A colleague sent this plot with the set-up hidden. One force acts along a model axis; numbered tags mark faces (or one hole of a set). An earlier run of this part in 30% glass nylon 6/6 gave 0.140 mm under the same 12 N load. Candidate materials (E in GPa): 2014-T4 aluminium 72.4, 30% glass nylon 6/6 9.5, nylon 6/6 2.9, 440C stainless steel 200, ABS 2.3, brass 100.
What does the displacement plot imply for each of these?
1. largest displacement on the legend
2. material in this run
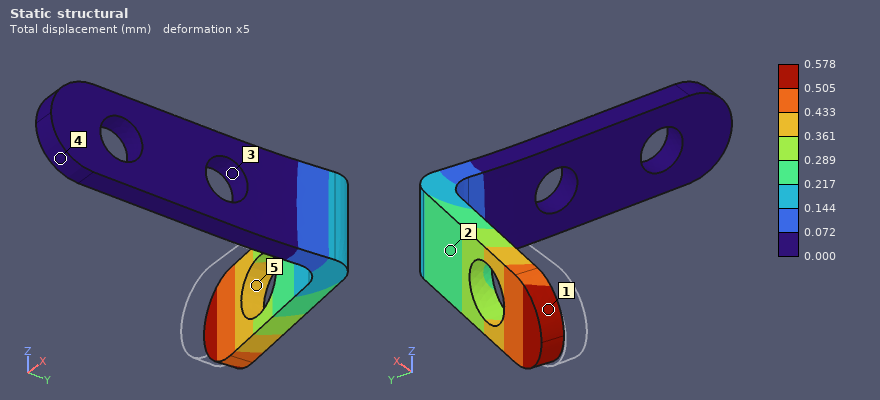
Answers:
0.578 mm
ABS
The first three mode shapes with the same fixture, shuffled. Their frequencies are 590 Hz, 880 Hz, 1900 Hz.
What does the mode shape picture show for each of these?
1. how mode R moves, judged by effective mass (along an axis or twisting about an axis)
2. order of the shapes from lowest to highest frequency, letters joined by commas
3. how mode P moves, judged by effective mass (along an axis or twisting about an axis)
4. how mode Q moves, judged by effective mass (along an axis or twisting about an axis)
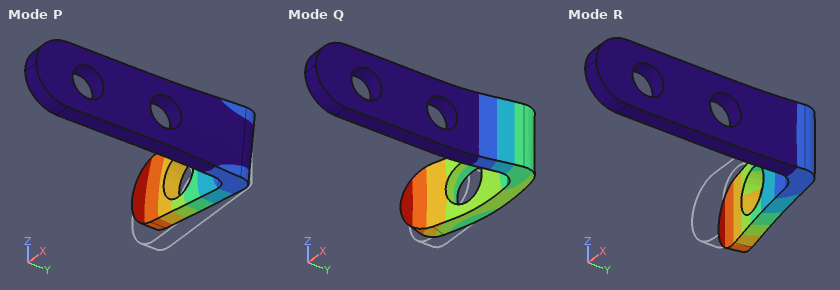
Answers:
along Y
R, P, Q
along Z
along X
